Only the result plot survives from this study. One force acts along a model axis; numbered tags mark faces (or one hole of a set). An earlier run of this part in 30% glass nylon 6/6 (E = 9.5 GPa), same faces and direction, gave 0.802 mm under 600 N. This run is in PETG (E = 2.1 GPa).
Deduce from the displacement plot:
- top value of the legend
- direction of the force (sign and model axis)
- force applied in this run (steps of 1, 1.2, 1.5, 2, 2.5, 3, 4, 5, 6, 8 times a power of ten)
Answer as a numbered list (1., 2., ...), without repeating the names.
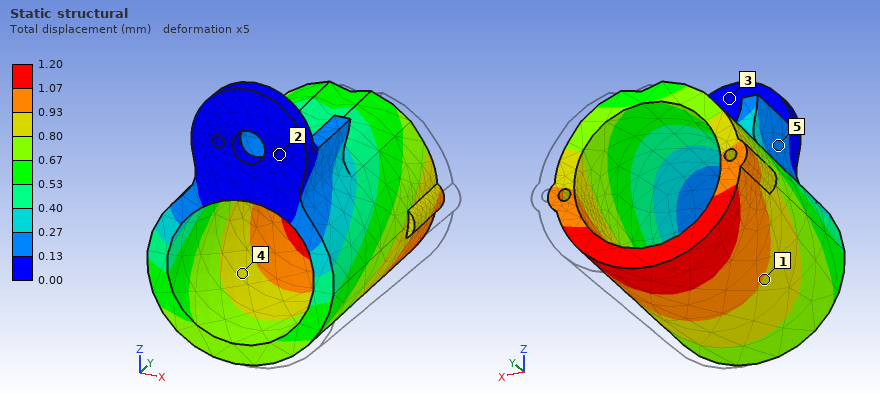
1. 1.20 mm
2. -X
3. 200 N
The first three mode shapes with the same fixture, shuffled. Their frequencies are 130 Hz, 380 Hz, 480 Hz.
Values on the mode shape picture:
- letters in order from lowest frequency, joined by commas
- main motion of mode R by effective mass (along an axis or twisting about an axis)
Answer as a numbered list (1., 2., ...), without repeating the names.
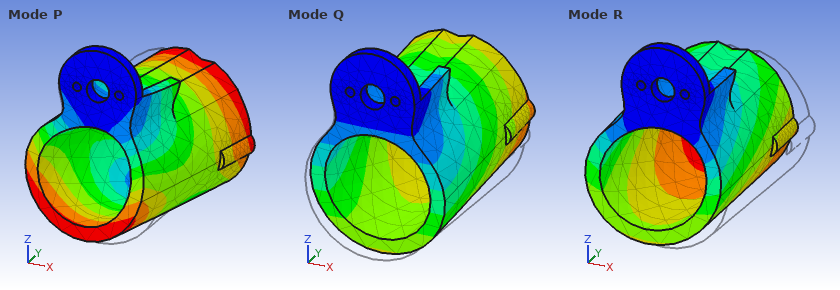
1. Q, R, P
2. along X
